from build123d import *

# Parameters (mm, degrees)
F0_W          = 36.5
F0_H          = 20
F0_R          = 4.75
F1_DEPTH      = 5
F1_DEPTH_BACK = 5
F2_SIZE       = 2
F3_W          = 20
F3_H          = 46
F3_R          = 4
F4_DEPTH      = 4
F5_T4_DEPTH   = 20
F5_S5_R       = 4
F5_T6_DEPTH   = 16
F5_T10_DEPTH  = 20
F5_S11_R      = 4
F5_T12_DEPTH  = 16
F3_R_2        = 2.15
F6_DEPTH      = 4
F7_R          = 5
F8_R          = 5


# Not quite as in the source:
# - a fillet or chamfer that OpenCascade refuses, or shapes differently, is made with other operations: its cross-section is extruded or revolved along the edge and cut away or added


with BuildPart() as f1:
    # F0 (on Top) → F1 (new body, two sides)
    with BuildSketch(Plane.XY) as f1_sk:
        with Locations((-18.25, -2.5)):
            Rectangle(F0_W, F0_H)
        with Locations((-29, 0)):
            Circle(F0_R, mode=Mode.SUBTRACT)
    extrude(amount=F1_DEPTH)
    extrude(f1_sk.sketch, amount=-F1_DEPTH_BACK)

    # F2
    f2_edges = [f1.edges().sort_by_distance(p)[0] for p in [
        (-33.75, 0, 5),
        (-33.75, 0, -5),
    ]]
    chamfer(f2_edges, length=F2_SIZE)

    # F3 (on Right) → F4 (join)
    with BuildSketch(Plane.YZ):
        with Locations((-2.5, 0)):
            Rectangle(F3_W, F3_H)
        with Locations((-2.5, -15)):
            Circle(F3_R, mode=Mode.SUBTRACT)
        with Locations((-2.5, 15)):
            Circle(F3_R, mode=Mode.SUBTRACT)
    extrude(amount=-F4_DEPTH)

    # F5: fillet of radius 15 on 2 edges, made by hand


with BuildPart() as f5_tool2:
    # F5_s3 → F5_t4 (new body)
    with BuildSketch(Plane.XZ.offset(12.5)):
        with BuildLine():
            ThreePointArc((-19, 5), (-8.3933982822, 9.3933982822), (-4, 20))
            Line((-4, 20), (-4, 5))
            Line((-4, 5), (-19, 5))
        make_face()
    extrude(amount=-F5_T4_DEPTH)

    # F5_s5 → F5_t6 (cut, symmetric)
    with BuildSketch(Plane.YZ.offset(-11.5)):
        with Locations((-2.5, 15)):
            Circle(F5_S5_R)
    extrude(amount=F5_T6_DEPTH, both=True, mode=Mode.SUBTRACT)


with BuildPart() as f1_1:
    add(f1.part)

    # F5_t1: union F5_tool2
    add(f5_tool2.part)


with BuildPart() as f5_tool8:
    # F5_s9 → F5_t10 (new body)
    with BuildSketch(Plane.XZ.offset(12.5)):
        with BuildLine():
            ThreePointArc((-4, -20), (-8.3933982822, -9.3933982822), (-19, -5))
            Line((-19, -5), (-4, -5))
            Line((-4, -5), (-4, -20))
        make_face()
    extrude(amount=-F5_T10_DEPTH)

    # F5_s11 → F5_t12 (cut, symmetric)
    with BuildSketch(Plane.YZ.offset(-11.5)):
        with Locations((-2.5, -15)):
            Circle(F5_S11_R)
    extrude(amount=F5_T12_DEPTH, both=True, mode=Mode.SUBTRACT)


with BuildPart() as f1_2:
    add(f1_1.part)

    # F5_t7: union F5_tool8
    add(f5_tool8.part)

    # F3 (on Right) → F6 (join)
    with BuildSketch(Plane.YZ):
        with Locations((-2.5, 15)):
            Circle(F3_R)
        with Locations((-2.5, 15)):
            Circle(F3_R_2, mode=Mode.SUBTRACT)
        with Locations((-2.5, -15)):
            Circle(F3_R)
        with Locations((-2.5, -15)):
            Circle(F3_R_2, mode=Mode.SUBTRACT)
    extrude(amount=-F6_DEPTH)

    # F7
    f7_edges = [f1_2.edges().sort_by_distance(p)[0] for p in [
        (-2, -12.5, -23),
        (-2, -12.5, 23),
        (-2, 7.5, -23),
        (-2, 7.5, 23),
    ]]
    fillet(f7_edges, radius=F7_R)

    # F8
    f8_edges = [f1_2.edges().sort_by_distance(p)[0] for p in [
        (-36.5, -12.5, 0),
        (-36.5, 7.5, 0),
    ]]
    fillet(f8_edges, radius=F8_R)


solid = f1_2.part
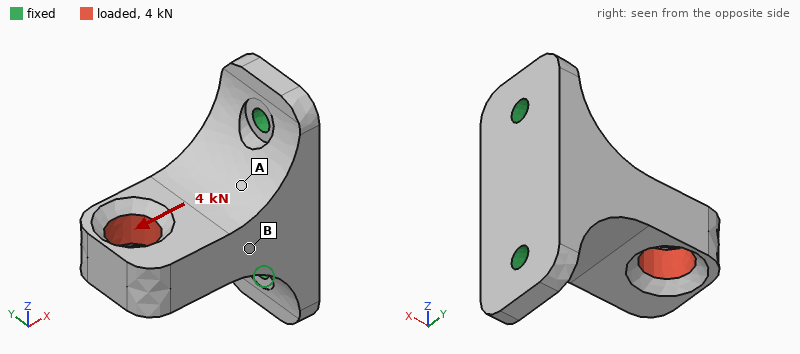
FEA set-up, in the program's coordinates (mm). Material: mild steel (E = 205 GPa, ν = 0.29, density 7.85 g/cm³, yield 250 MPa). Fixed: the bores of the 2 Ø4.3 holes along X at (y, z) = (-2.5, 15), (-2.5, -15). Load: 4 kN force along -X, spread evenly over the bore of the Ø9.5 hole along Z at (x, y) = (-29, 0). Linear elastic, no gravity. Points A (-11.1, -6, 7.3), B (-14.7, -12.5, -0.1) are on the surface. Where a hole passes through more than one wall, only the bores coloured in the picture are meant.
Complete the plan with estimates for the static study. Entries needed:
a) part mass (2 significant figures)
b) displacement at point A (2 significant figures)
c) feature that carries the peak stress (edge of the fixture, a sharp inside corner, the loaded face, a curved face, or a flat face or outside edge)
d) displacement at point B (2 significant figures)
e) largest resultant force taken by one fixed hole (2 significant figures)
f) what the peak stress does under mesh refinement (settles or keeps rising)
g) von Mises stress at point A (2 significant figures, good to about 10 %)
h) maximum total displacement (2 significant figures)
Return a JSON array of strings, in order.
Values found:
["85 g", "5.5 µm", "edge of the fixture", "7.2 µm", "2.3 kN", "keeps rising", "31 MPa", "27 µm"]
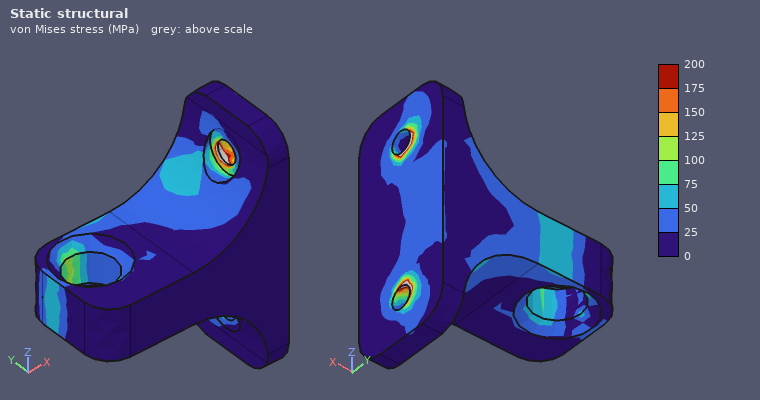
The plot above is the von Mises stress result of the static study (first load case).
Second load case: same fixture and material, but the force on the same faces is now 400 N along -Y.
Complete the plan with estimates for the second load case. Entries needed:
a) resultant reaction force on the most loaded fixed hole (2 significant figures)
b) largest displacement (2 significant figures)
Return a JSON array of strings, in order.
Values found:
["200 N", "25 µm"]
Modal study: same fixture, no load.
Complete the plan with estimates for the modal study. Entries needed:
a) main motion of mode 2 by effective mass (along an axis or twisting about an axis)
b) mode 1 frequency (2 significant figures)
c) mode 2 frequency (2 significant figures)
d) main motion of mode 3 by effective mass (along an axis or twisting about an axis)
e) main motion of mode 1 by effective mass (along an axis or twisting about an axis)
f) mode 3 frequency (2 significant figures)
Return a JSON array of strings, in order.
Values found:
["along Z", "4600 Hz", "11 kHz", "along X", "along Y", "18 kHz"]
